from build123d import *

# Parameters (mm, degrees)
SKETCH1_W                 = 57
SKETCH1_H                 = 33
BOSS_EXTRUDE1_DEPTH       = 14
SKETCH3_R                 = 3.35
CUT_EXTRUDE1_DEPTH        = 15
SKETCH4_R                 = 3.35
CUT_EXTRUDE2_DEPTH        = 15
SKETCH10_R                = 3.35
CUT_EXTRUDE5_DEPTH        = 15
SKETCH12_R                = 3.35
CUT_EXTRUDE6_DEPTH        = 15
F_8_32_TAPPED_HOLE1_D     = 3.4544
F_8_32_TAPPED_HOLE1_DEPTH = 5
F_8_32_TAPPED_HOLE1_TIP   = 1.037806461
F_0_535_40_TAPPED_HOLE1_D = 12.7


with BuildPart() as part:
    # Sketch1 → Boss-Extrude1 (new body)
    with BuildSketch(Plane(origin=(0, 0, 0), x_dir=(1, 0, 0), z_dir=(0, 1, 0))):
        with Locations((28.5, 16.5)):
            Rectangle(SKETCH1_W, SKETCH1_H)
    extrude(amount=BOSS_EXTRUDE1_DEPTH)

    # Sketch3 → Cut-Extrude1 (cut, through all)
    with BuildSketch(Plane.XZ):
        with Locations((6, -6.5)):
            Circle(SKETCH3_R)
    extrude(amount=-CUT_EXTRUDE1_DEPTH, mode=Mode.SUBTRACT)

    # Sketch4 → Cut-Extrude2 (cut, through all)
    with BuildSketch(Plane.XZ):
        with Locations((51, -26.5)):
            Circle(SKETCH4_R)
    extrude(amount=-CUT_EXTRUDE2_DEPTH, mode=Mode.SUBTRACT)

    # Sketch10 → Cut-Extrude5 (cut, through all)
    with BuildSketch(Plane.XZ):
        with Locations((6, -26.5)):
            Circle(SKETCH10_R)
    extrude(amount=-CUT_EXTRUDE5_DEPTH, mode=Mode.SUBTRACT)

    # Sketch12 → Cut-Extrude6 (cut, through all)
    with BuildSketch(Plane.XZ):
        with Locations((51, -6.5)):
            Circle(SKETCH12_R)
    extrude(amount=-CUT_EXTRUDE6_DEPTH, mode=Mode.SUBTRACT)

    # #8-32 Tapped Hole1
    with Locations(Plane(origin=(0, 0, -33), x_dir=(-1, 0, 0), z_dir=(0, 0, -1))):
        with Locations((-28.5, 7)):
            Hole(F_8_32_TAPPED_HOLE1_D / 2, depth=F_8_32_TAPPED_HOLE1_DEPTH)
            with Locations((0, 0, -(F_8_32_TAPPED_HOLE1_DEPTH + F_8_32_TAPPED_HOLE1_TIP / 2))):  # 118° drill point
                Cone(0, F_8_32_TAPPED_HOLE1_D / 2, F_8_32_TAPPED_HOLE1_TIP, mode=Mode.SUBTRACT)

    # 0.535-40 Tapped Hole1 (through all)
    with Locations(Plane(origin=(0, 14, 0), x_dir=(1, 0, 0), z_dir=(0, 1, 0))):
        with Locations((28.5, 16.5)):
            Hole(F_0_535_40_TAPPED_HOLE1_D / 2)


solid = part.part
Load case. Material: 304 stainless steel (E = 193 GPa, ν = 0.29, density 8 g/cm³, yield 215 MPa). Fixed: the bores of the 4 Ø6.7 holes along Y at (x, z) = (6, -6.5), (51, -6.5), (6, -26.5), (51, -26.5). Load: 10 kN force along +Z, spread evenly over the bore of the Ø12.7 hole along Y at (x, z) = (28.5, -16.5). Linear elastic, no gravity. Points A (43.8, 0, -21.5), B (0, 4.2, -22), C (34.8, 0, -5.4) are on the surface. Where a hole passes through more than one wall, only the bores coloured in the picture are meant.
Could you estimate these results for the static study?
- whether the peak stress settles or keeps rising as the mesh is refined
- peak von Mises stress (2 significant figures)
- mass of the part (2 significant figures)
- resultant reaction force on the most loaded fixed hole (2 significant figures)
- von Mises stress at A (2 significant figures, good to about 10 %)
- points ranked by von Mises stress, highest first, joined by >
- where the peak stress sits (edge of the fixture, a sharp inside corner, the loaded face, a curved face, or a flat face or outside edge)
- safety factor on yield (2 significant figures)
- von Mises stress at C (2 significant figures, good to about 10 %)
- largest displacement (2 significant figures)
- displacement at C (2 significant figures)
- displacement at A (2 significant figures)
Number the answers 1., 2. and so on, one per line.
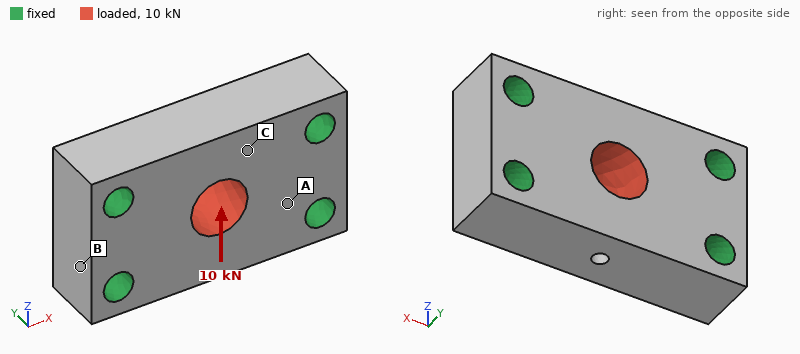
1. settles
2. 59 MPa
3. 180 g
4. 3.2 kN
5. 25 MPa
6. A > C > B
7. a curved face
8. 3.7
9. 17 MPa
10. 3.9 µm
11. 2.8 µm
12. 0.99 µm
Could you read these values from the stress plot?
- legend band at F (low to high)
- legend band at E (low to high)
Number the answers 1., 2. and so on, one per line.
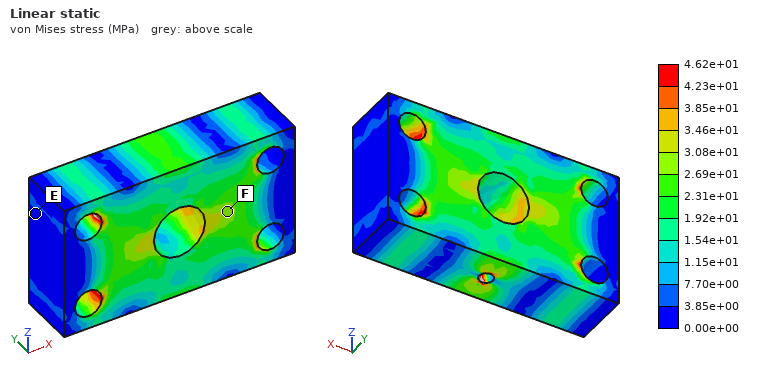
1. 2.69e+01 to 3.08e+01 MPa
2. 0.00e+00 to 3.85e+00 MPa
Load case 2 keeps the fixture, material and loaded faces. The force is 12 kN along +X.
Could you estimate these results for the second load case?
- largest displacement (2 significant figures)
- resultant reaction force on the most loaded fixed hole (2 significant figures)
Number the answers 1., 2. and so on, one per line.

1. 1.8 µm
2. 3.1 kN
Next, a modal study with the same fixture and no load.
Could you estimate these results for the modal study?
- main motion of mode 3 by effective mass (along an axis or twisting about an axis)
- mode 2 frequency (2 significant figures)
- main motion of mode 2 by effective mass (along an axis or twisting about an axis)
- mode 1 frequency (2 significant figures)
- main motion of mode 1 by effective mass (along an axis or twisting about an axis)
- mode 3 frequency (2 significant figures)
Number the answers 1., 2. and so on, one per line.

1. along Z
2. 31 kHz
3. twisting about X
4. 27 kHz
5. along Y
6. 34 kHz
